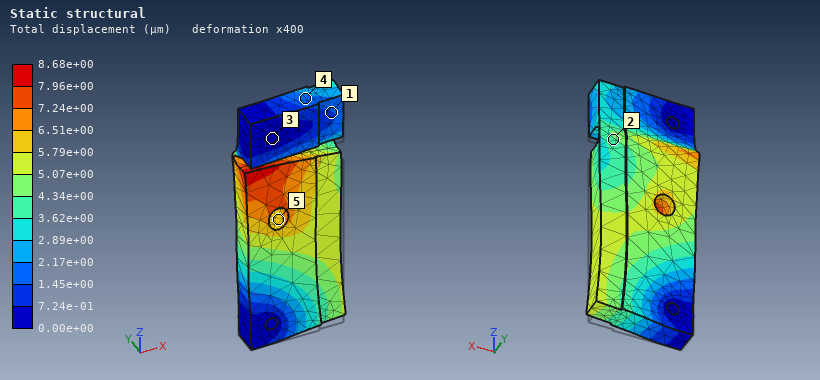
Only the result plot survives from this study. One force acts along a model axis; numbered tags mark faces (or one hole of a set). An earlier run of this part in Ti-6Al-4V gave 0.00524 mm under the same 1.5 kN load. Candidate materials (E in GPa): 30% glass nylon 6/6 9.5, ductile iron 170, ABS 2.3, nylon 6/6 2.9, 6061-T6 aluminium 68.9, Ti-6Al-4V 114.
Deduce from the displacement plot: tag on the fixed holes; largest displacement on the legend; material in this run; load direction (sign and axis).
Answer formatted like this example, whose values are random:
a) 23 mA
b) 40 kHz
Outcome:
a) 3
b) 8.68e+00 µm
c) 6061-T6 aluminium
d) +Z
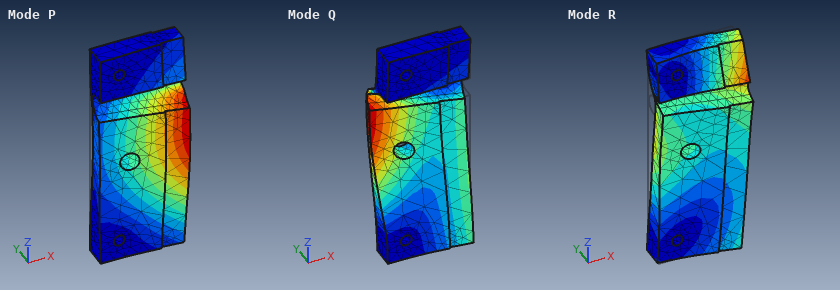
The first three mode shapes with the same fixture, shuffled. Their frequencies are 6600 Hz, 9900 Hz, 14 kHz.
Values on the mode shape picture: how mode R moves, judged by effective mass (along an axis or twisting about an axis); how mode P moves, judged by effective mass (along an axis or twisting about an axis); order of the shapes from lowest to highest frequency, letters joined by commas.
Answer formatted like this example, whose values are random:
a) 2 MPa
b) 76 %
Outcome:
a) along X
b) along Y
c) P, Q, R
